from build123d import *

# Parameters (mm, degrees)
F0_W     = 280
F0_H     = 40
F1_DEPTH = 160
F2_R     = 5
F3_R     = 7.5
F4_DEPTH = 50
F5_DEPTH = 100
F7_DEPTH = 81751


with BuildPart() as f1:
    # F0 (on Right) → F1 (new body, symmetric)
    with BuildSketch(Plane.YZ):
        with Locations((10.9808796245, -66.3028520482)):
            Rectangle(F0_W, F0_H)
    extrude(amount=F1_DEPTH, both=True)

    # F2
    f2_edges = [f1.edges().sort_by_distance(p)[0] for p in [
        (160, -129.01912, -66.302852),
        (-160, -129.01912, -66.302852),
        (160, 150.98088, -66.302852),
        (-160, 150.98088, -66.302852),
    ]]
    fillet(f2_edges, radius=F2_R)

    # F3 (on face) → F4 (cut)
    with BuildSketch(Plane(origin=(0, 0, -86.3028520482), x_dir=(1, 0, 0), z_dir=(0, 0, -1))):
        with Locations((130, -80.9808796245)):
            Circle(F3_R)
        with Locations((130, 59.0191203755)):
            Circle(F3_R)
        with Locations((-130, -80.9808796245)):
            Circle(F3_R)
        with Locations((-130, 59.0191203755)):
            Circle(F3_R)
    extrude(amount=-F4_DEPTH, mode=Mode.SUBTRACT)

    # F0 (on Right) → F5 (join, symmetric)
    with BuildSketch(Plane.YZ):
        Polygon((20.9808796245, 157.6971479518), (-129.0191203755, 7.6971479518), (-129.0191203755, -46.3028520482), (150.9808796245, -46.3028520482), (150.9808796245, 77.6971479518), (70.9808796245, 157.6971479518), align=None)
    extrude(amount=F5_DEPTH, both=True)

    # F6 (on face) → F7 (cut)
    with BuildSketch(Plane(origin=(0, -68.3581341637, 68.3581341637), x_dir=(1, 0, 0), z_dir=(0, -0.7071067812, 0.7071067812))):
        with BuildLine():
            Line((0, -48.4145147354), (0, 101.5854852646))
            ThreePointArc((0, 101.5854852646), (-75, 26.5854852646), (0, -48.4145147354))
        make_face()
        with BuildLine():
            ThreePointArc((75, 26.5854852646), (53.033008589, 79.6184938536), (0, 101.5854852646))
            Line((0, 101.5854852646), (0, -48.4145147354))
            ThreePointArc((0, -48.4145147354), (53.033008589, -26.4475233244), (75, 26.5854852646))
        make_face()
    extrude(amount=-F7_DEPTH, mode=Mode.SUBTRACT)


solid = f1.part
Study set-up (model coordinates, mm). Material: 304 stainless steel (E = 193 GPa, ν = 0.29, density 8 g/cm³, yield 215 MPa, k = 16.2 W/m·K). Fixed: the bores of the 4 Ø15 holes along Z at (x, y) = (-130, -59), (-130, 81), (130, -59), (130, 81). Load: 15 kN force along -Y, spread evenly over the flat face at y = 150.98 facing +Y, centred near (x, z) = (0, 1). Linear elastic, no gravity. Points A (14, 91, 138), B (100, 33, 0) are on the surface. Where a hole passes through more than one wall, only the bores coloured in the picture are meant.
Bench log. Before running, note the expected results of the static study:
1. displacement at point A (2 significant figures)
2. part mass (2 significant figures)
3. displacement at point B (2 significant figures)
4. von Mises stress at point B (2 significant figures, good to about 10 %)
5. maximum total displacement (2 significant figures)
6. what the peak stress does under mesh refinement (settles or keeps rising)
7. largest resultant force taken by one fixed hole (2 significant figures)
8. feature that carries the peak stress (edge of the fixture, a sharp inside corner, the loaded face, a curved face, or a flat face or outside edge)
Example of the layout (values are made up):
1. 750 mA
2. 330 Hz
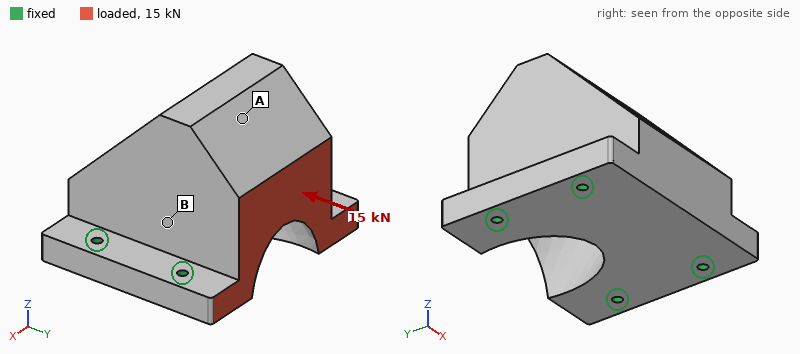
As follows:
1. 6.0 µm
2. 64 kg
3. 2.5 µm
4. 1.5 MPa
5. 6.3 µm
6. keeps rising
7. 5.4 kN
8. edge of the fixture
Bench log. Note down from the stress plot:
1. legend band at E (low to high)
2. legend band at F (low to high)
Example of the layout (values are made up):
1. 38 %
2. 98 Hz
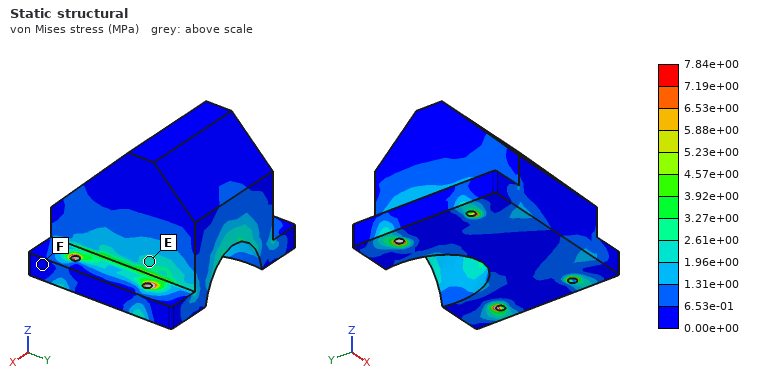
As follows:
1. 1.96e+00 to 2.61e+00 MPa
2. 0.00e+00 to 6.53e-01 MPa
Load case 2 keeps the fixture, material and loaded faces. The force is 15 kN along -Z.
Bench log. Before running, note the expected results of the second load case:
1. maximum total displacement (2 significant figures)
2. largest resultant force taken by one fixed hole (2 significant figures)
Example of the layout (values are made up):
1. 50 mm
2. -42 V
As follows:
1. 9.8 µm
2. 10 kN
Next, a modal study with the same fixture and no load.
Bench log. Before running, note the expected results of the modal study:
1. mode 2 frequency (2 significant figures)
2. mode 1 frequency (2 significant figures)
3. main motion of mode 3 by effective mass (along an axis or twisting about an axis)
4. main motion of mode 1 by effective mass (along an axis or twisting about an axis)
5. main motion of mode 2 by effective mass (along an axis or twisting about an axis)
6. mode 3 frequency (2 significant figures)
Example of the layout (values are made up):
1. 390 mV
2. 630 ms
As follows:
1. 1400 Hz
2. 1100 Hz
3. along Z
4. along Y
5. along X
6. 2000 Hz
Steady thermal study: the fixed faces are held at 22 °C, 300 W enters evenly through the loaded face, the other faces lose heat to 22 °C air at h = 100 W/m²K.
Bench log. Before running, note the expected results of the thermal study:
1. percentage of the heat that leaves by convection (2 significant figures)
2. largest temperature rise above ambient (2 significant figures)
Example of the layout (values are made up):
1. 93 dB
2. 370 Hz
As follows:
1. 89 %
2. 59 K
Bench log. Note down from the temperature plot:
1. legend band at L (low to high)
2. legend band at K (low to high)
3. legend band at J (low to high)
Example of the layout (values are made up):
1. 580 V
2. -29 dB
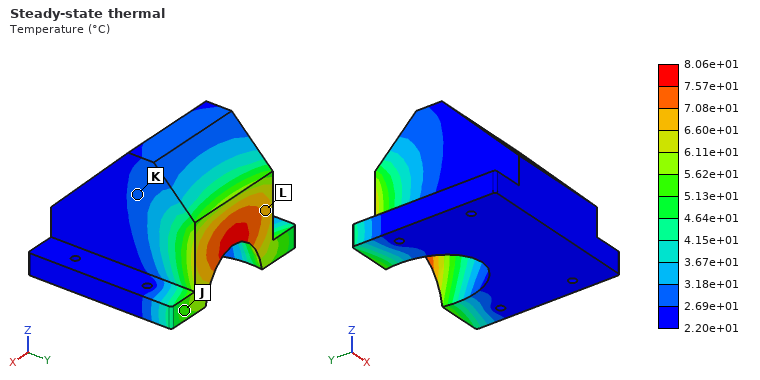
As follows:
1. 6.60e+01 to 7.08e+01 °C
2. 2.69e+01 to 3.18e+01 °C
3. 5.13e+01 to 5.62e+01 °C
